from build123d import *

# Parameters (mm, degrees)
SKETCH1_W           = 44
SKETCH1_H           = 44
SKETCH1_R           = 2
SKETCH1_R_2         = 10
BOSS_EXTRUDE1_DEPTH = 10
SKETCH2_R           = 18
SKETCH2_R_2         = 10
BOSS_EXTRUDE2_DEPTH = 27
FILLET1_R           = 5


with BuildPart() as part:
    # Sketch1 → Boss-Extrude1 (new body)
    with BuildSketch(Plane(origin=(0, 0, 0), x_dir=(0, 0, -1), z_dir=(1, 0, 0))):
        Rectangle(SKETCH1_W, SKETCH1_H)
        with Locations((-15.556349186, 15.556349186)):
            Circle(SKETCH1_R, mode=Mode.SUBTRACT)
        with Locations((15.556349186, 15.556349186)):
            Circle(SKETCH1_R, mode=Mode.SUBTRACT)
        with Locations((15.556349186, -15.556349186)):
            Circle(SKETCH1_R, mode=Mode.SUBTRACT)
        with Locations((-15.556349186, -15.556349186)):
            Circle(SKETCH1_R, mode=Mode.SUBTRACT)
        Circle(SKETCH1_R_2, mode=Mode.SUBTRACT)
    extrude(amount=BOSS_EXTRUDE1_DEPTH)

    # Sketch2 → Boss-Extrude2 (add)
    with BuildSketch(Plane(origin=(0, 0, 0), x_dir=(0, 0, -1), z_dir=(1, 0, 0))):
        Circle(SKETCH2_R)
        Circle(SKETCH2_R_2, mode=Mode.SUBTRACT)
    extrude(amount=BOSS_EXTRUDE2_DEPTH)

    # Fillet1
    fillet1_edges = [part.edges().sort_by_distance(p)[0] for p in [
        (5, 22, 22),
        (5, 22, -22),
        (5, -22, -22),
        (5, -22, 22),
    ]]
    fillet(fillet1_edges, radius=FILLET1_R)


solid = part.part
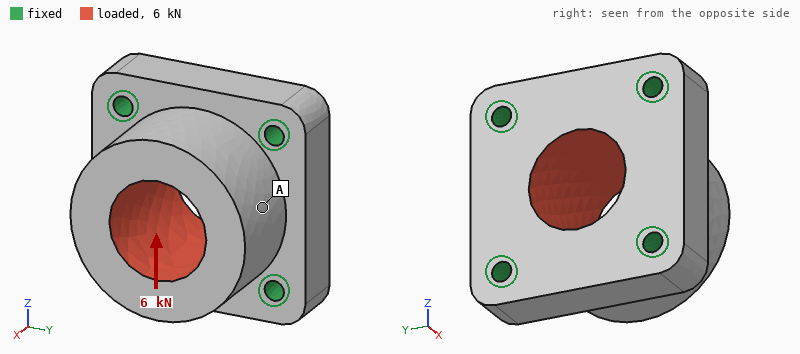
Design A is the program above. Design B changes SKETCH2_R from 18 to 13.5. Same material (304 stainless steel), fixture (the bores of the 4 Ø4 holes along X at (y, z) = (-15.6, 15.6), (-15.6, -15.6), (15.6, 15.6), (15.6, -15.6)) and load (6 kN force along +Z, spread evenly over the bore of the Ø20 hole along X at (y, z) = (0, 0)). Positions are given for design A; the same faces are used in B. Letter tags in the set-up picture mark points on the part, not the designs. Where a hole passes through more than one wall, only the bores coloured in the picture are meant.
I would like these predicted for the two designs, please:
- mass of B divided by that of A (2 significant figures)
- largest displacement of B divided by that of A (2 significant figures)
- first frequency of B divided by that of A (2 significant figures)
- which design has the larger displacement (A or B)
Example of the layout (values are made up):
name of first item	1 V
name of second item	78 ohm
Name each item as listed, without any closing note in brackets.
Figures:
mass of B divided by that of A	0.72
largest displacement of B divided by that of A	2.5
first frequency of B divided by that of A	1.0
which design has the larger displacement	B
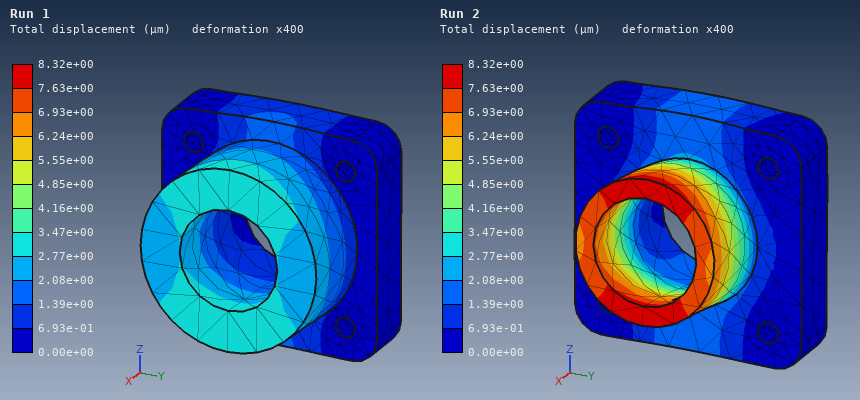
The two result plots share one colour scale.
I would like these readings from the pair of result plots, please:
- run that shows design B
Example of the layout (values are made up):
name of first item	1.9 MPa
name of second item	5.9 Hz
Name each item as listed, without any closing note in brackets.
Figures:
run that shows design B	Run 2
